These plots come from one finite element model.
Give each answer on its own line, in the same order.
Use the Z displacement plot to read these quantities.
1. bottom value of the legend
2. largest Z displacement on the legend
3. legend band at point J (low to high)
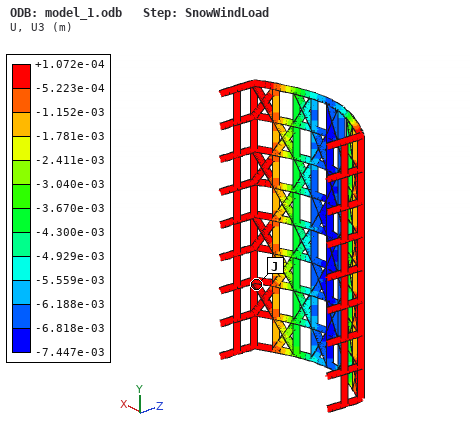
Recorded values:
-7.447e-03 m
+1.072e-04 m
-5.223e-04 to +1.072e-04 m
